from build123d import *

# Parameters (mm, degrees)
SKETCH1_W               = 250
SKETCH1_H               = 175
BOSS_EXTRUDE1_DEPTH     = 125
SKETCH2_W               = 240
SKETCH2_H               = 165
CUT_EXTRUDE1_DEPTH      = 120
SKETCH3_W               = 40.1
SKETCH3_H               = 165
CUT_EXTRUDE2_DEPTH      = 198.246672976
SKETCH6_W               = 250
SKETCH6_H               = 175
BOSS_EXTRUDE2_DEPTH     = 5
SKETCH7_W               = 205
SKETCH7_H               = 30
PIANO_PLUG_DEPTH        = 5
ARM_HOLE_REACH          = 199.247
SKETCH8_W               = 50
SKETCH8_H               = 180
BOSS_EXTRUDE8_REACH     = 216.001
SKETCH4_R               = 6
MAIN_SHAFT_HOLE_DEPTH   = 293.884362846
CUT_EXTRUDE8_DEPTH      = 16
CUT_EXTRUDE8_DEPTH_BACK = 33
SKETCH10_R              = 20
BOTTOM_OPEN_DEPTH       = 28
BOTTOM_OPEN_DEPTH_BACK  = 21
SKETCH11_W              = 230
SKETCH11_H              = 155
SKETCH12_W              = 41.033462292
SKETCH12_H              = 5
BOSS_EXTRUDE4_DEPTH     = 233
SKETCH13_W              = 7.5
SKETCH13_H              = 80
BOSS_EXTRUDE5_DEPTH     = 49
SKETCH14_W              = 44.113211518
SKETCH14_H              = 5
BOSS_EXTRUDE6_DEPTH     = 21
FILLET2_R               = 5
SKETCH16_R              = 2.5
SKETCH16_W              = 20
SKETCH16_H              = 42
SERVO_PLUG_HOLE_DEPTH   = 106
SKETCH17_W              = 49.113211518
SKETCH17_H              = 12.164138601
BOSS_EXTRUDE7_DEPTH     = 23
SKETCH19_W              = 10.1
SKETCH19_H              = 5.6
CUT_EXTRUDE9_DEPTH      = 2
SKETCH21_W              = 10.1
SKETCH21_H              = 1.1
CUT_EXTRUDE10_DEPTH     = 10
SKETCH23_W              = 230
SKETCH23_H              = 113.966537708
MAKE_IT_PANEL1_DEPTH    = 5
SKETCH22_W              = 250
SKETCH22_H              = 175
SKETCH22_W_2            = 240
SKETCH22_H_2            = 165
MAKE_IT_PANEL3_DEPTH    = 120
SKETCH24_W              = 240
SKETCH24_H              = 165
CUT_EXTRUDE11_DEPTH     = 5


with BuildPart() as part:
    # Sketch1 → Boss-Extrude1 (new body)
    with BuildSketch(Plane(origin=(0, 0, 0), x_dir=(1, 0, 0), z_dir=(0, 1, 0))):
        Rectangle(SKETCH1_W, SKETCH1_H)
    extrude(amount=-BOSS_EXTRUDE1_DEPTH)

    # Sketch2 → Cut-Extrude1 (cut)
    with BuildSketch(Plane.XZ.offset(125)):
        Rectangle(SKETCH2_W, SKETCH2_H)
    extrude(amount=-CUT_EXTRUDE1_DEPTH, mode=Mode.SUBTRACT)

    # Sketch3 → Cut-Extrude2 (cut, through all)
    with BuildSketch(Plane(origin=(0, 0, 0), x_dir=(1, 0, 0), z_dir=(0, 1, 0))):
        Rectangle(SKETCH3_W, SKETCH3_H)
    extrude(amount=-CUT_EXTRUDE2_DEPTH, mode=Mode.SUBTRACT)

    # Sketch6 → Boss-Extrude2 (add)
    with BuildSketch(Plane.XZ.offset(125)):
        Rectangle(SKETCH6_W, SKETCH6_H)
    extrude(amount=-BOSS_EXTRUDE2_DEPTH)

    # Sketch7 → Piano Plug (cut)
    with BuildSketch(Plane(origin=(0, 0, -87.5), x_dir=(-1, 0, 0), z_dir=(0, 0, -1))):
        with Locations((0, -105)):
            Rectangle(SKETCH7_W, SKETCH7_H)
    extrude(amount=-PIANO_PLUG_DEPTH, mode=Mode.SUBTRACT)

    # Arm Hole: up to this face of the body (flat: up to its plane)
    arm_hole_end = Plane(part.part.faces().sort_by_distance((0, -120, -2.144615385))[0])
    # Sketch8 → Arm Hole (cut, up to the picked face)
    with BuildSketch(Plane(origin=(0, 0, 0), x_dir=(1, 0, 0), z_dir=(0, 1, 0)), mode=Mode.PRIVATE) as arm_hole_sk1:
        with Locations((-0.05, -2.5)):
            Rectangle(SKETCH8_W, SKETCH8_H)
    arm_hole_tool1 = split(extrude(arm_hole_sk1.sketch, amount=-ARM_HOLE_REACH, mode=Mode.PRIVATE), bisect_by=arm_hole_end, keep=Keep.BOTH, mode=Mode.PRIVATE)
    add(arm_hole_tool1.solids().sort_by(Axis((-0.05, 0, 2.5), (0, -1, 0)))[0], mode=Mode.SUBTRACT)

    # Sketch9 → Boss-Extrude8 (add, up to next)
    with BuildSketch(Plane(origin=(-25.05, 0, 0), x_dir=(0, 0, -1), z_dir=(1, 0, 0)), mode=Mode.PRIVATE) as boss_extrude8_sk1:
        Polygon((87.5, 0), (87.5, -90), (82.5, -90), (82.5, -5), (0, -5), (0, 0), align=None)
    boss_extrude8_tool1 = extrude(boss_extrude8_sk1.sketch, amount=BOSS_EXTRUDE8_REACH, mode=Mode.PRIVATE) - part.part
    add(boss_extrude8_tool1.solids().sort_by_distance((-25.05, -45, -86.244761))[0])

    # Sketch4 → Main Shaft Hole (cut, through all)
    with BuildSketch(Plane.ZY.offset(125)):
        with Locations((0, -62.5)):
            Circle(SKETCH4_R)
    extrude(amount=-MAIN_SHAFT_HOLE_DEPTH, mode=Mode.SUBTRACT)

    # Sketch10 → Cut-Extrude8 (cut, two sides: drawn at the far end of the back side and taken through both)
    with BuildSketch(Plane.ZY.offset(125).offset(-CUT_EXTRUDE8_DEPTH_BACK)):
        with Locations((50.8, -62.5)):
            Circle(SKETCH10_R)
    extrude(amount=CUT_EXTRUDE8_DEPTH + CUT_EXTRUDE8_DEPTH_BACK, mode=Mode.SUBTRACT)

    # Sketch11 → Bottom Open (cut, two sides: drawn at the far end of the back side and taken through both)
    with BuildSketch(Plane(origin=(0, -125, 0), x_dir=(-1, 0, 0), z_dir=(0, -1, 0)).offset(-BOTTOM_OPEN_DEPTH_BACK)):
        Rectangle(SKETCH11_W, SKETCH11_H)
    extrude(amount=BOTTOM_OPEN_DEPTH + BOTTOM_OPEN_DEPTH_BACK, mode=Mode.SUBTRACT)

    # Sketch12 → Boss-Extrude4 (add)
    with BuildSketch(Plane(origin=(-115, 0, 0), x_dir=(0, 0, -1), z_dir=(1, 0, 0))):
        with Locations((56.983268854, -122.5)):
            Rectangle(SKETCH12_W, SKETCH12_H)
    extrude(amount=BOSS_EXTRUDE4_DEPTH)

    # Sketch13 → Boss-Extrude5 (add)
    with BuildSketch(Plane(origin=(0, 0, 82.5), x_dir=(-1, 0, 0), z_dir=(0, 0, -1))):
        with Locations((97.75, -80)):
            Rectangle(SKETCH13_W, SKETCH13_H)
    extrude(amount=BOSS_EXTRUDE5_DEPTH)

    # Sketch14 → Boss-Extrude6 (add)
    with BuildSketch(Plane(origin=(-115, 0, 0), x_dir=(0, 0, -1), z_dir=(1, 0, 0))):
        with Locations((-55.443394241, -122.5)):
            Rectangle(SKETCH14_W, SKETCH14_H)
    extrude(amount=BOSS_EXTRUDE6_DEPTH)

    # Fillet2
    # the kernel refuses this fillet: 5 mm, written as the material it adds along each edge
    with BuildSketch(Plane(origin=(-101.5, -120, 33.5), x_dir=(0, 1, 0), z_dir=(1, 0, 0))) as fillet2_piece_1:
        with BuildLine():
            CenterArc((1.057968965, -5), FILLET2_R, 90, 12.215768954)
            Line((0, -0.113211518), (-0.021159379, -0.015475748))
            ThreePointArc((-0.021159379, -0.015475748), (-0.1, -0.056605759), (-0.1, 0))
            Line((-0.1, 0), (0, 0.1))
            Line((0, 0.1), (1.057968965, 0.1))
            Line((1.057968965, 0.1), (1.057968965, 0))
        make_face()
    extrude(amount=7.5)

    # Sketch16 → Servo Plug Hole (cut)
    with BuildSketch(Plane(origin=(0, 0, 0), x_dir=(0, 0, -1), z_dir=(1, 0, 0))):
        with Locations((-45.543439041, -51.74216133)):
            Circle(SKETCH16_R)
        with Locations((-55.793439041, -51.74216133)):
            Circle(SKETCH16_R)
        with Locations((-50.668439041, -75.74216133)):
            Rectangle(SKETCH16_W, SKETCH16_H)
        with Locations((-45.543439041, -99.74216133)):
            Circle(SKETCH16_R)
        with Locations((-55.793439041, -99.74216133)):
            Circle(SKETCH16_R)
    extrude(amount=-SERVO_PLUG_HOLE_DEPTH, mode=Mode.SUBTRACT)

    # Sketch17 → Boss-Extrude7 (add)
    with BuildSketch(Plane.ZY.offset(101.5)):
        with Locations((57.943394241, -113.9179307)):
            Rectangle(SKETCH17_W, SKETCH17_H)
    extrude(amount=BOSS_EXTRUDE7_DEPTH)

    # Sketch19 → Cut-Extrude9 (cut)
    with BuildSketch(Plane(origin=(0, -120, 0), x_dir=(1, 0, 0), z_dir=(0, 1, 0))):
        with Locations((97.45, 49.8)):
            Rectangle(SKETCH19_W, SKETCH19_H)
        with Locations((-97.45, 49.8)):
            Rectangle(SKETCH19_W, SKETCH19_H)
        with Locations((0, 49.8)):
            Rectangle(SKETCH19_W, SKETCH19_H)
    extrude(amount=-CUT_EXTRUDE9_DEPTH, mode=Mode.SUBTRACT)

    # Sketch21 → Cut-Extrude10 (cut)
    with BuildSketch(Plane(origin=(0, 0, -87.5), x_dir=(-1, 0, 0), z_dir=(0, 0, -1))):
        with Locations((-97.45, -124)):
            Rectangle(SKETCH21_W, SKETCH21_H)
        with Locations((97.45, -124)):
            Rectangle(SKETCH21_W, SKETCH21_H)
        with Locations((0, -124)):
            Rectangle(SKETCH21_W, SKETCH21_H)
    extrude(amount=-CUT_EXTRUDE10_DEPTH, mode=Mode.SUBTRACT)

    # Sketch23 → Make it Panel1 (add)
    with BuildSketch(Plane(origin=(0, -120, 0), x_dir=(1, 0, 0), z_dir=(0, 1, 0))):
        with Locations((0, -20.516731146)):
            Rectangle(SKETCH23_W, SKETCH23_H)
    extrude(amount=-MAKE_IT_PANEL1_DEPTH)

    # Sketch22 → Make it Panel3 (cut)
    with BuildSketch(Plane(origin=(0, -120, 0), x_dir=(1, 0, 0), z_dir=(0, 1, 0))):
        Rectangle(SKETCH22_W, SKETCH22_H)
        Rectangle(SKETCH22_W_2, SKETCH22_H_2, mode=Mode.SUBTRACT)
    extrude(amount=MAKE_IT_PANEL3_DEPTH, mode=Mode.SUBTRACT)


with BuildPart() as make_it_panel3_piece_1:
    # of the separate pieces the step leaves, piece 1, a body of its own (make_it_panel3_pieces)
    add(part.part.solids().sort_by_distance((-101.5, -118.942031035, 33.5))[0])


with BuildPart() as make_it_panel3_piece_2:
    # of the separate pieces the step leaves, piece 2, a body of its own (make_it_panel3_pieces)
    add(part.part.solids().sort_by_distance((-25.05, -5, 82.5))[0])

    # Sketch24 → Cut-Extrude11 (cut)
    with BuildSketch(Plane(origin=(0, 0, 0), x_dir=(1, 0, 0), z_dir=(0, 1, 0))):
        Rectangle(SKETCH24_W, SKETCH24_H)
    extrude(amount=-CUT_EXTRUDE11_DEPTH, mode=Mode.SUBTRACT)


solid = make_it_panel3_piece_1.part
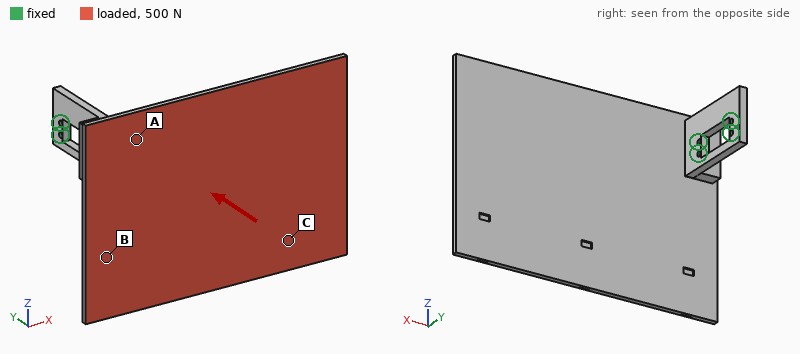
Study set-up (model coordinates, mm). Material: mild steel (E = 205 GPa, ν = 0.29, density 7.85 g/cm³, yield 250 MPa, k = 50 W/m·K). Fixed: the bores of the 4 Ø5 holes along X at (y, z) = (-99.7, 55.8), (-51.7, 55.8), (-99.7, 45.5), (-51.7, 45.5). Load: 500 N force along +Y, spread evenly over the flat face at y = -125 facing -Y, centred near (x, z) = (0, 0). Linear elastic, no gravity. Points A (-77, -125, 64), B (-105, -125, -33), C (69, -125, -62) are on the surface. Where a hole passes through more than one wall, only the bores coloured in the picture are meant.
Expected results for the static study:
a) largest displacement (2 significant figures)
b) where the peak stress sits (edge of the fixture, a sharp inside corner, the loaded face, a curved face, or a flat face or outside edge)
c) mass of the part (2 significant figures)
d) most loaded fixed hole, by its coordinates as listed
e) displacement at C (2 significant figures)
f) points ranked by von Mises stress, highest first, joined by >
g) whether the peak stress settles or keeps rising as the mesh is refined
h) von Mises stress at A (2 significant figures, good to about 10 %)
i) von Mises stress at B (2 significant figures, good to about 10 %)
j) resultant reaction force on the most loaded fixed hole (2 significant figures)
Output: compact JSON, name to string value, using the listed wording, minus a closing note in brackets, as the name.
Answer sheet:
{"largest displacement": "3.2 mm", "where the peak stress sits": "a sharp inside corner", "mass of the part": "2.0 kg", "most loaded fixed hole, by its coordinates as listed": "(-99.7, 45.5)", "displacement at C": "2.3 mm", "points ranked by von Mises stress, highest first, joined by >": "A > B > C", "whether the peak stress settles or keeps rising as the mesh is refined": "keeps rising", "von Mises stress at A": "91 MPa", "von Mises stress at B": "34 MPa", "resultant reaction force on the most loaded fixed hole": "1.2 kN"}
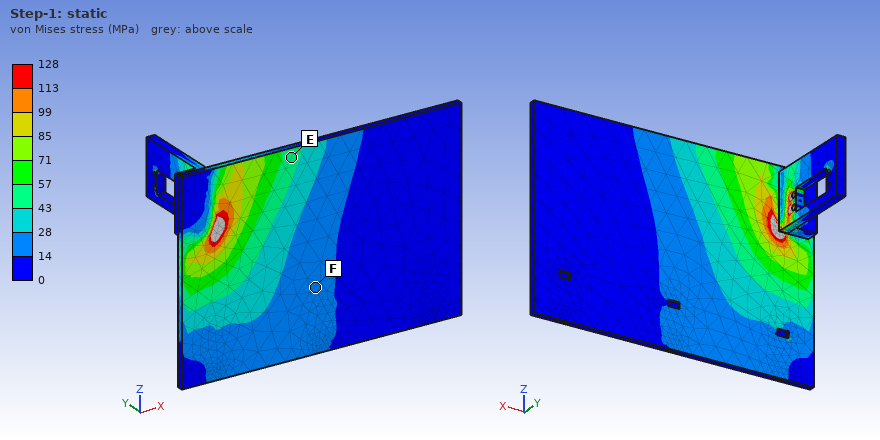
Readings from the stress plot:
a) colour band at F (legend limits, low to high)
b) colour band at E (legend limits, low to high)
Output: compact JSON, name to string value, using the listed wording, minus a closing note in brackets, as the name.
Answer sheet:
{"colour band at F": "14 to 28 MPa", "colour band at E": "43 to 57 MPa"}
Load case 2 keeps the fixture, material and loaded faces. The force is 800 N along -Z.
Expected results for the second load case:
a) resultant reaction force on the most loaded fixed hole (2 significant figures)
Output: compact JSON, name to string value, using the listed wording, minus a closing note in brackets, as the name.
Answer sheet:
{"resultant reaction force on the most loaded fixed hole": "3.5 kN"}
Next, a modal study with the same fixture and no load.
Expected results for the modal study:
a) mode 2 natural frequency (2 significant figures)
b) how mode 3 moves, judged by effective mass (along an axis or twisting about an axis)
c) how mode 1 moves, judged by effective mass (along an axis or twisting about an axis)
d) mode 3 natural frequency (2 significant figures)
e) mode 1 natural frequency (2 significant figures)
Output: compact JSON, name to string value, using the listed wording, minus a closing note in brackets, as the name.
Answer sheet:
{"mode 2 natural frequency": "170 Hz", "how mode 3 moves, judged by effective mass": "along Z", "how mode 1 moves, judged by effective mass": "along Y", "mode 3 natural frequency": "210 Hz", "mode 1 natural frequency": "63 Hz"}
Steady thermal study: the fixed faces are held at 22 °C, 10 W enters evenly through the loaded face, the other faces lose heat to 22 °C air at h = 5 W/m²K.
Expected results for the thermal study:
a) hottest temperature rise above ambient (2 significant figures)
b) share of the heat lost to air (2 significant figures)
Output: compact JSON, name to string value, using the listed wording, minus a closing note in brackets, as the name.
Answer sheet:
{"hottest temperature rise above ambient": "23 K", "share of the heat lost to air": "46 %"}
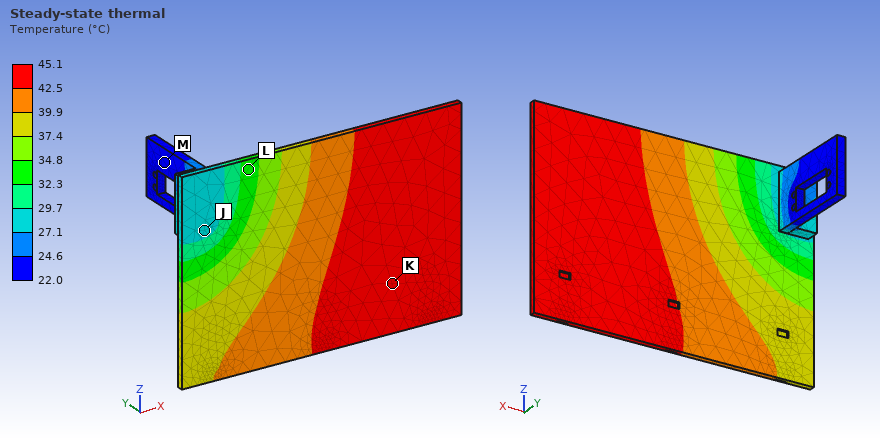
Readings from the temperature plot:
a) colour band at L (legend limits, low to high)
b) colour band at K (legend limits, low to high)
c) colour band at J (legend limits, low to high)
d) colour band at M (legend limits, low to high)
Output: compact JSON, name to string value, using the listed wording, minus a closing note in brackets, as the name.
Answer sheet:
{"colour band at L": "32.3 to 34.8 °C", "colour band at K": "42.5 to 45.1 °C", "colour band at J": "27.1 to 29.7 °C", "colour band at M": "22.0 to 24.6 °C"}
